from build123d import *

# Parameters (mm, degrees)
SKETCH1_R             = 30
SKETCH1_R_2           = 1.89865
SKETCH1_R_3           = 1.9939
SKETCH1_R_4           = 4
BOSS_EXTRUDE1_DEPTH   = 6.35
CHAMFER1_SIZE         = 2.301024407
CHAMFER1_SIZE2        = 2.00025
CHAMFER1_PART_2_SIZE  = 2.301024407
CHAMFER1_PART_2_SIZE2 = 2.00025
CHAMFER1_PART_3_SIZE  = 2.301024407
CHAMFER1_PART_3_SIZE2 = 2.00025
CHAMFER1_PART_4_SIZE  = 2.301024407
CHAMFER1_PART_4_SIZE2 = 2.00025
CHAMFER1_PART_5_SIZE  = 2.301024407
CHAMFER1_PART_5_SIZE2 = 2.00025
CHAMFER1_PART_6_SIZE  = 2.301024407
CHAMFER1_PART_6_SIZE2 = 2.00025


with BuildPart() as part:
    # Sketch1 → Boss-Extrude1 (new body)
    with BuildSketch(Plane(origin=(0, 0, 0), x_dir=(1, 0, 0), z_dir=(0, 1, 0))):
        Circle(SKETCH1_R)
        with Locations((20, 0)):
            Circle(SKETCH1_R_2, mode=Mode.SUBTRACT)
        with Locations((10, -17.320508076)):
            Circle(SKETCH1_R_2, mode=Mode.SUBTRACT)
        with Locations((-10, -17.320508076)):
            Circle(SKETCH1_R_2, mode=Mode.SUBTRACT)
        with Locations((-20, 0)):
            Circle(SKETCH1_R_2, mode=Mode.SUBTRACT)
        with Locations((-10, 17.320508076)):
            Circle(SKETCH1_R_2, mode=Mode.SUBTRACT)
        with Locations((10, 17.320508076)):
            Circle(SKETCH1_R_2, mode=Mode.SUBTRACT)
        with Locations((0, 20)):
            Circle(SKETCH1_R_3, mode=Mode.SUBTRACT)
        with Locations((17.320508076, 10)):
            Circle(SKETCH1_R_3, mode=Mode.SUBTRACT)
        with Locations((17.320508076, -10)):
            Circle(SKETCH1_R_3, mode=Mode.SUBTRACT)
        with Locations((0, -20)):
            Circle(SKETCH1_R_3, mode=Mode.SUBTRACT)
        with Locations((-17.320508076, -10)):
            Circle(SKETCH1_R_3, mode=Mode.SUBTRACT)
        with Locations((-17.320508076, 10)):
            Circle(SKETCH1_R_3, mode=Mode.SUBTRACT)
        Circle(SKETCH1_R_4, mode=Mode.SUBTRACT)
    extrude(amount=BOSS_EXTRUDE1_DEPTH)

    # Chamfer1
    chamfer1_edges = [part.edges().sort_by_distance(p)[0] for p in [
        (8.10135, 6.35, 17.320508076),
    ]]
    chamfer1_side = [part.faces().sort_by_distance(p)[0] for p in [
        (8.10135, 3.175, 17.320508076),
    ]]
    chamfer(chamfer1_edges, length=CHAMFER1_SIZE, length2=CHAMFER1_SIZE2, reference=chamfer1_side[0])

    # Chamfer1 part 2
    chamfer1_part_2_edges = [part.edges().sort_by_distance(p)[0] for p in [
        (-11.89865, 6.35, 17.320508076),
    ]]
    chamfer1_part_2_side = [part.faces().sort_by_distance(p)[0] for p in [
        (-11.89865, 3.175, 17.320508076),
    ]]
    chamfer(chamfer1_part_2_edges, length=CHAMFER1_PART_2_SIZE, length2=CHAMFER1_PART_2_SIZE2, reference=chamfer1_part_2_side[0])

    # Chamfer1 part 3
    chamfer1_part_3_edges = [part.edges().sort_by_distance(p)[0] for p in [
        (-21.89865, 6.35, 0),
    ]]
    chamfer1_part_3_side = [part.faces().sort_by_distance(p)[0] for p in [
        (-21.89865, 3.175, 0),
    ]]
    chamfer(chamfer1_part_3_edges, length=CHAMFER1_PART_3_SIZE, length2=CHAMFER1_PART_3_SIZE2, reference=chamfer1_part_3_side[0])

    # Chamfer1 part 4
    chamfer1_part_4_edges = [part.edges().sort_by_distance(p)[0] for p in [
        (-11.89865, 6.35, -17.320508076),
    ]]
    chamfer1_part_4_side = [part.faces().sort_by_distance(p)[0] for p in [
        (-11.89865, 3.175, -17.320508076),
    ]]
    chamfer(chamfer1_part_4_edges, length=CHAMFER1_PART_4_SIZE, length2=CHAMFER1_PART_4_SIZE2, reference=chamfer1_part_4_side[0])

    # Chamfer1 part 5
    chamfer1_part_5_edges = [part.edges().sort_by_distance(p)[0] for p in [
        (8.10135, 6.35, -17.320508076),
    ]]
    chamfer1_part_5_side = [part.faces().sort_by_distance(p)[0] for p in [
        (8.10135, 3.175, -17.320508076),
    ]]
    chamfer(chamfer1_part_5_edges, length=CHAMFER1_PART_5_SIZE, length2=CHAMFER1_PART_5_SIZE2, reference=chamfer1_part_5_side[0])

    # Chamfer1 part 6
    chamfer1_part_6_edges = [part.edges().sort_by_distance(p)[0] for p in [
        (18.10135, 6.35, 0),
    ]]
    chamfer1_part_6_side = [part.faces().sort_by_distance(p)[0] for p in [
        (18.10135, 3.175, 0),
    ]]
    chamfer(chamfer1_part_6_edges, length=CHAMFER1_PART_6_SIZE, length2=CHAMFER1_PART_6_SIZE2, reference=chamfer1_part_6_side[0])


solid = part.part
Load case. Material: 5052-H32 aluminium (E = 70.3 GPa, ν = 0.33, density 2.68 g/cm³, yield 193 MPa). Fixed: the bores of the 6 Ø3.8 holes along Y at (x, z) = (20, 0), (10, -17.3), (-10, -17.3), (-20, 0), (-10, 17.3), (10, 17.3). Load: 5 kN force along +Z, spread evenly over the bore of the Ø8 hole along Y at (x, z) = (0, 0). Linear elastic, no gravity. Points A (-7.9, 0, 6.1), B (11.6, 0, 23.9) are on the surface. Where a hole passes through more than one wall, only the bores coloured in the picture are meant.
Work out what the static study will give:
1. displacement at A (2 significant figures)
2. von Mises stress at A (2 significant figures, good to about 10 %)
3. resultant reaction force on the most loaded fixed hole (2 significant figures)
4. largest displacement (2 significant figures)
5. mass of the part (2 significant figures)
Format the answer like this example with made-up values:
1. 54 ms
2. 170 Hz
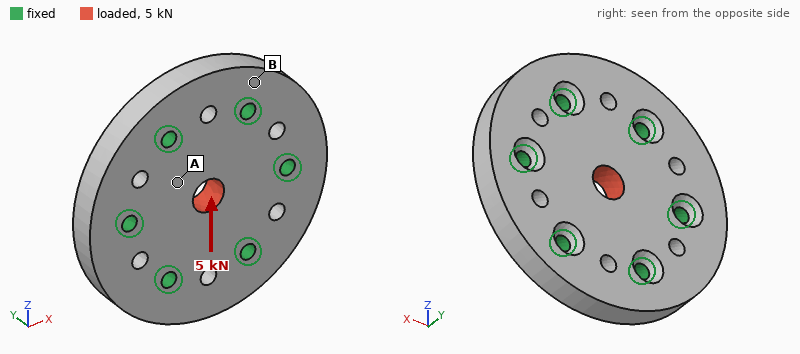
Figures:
1. 2.6 µm
2. 17 MPa
3. 1.1 kN
4. 5.6 µm
5. 44 g
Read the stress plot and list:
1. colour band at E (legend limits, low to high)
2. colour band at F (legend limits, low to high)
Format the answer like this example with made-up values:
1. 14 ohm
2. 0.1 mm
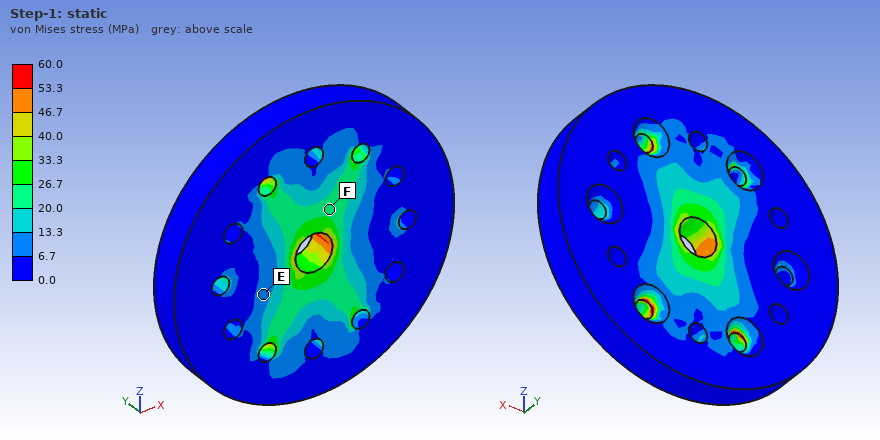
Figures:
1. 6.7 to 13.3 MPa
2. 20.0 to 26.7 MPa
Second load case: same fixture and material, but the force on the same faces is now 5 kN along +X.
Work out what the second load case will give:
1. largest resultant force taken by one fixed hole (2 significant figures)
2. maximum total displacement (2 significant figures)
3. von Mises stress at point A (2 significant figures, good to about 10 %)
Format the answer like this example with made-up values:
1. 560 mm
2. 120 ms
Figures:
1. 1.3 kN
2. 5.6 µm
3. 17 MPa
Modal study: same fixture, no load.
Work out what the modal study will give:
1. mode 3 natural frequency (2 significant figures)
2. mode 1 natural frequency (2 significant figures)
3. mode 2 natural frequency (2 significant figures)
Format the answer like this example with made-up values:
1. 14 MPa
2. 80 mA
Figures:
1. 25 kHz
2. 23 kHz
3. 25 kHz
